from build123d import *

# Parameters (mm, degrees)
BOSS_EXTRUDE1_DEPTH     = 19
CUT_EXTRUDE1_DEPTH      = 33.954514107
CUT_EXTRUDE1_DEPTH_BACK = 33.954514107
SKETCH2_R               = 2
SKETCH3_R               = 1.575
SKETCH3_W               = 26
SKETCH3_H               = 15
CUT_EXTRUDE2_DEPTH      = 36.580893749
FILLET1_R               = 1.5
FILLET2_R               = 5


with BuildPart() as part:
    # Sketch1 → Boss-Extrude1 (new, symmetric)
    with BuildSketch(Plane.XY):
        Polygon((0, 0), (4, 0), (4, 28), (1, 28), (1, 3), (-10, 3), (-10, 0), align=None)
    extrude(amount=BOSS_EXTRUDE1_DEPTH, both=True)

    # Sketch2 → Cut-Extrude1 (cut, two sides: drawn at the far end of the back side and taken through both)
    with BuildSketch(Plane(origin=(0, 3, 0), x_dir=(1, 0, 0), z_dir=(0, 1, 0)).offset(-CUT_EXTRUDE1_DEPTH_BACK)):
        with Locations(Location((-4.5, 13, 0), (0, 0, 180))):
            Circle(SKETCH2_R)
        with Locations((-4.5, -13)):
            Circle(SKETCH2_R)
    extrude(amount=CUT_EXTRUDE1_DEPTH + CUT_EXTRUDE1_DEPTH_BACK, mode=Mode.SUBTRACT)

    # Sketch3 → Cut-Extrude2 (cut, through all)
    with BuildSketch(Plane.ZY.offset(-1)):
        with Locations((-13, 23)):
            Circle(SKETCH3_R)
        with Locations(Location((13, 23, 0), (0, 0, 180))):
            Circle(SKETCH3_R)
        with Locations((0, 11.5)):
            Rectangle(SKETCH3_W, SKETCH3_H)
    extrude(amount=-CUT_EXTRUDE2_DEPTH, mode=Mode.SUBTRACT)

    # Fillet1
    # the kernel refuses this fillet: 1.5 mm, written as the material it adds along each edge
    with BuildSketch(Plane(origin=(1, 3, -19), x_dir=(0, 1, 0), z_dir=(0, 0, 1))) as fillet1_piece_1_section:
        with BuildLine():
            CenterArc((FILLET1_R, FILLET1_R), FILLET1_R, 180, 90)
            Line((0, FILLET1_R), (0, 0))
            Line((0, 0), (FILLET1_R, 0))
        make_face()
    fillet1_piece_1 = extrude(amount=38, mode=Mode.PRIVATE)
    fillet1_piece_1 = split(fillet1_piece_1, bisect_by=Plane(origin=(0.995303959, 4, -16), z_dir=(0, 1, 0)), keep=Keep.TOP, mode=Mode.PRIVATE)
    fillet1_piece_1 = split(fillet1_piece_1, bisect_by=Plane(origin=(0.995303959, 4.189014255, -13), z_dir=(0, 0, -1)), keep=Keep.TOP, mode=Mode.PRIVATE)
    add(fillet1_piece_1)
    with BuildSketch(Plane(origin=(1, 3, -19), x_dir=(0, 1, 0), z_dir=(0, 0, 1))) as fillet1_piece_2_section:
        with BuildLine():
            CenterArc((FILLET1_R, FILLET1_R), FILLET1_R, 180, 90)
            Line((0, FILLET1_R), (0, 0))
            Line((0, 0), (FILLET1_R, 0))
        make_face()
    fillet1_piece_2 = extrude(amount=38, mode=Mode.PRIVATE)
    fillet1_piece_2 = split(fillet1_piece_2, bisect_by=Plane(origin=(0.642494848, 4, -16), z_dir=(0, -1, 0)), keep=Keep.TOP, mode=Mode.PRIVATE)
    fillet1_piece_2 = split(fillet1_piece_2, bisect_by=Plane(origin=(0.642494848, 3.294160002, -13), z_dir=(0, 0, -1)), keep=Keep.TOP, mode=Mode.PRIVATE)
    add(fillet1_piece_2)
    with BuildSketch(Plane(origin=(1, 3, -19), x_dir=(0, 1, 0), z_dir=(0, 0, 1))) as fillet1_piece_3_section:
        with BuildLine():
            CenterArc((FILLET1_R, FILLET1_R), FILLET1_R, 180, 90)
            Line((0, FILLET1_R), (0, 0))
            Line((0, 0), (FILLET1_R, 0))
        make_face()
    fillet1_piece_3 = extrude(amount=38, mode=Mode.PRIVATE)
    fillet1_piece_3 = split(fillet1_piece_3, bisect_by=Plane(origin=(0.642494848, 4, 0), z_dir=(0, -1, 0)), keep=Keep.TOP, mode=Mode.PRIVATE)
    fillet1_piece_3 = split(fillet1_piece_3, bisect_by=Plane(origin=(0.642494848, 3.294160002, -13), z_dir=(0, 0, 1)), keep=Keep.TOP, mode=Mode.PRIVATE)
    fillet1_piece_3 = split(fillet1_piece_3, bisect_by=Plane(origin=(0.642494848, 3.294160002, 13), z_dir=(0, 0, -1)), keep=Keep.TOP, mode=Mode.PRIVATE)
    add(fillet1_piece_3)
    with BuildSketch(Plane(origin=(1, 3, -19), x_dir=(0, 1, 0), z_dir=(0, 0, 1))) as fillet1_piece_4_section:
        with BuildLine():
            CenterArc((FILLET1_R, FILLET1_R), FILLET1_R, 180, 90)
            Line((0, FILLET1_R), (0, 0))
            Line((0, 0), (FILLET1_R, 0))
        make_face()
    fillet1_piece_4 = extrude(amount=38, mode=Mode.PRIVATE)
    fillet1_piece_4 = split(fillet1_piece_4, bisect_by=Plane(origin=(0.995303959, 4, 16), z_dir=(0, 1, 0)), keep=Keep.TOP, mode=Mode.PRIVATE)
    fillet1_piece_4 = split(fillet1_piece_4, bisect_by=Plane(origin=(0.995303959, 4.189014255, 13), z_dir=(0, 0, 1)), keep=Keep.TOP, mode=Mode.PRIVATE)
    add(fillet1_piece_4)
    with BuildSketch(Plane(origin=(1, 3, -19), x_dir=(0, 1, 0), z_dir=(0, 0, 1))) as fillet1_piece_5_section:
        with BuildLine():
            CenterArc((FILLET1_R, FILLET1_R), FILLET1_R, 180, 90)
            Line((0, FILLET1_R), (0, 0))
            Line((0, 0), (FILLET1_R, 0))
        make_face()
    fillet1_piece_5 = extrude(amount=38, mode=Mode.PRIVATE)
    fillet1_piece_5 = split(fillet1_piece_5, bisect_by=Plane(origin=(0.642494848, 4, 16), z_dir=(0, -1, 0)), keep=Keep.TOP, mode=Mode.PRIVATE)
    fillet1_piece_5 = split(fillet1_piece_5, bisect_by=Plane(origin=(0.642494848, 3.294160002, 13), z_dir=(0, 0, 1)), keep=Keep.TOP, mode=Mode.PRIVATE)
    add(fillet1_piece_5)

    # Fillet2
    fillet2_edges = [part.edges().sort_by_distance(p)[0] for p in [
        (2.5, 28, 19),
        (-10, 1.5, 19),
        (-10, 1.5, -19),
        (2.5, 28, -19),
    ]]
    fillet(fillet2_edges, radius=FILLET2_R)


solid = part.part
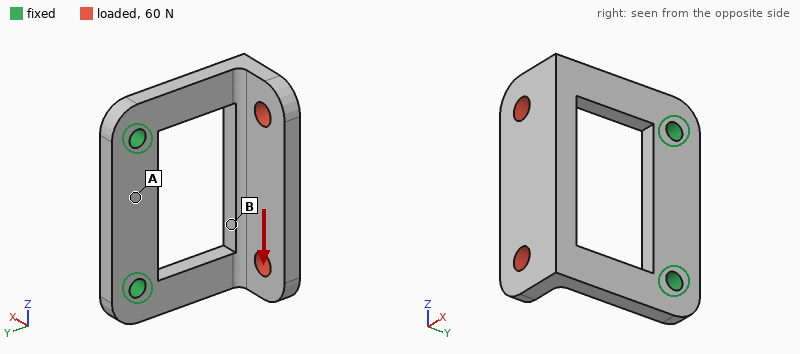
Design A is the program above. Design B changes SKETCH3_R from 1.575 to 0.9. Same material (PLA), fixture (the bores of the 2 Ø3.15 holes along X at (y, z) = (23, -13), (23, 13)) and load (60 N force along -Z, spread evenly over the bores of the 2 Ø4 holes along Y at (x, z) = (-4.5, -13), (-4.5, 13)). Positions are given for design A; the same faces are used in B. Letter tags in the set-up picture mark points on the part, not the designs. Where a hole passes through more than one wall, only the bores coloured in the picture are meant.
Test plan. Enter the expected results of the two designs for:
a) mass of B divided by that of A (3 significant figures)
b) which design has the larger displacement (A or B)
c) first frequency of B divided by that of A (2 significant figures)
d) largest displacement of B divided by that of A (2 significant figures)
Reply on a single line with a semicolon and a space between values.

1.01; B; 0.95; 1.1
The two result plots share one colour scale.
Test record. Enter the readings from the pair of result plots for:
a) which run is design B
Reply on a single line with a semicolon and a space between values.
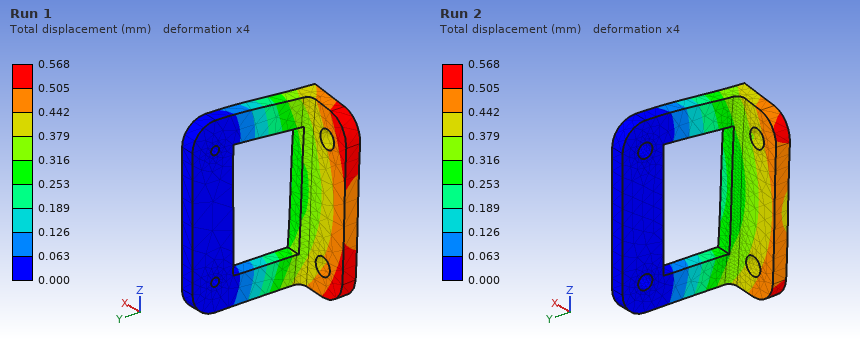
Run 1
